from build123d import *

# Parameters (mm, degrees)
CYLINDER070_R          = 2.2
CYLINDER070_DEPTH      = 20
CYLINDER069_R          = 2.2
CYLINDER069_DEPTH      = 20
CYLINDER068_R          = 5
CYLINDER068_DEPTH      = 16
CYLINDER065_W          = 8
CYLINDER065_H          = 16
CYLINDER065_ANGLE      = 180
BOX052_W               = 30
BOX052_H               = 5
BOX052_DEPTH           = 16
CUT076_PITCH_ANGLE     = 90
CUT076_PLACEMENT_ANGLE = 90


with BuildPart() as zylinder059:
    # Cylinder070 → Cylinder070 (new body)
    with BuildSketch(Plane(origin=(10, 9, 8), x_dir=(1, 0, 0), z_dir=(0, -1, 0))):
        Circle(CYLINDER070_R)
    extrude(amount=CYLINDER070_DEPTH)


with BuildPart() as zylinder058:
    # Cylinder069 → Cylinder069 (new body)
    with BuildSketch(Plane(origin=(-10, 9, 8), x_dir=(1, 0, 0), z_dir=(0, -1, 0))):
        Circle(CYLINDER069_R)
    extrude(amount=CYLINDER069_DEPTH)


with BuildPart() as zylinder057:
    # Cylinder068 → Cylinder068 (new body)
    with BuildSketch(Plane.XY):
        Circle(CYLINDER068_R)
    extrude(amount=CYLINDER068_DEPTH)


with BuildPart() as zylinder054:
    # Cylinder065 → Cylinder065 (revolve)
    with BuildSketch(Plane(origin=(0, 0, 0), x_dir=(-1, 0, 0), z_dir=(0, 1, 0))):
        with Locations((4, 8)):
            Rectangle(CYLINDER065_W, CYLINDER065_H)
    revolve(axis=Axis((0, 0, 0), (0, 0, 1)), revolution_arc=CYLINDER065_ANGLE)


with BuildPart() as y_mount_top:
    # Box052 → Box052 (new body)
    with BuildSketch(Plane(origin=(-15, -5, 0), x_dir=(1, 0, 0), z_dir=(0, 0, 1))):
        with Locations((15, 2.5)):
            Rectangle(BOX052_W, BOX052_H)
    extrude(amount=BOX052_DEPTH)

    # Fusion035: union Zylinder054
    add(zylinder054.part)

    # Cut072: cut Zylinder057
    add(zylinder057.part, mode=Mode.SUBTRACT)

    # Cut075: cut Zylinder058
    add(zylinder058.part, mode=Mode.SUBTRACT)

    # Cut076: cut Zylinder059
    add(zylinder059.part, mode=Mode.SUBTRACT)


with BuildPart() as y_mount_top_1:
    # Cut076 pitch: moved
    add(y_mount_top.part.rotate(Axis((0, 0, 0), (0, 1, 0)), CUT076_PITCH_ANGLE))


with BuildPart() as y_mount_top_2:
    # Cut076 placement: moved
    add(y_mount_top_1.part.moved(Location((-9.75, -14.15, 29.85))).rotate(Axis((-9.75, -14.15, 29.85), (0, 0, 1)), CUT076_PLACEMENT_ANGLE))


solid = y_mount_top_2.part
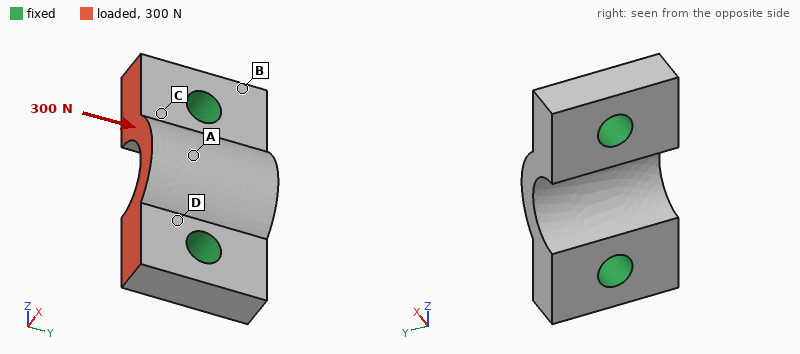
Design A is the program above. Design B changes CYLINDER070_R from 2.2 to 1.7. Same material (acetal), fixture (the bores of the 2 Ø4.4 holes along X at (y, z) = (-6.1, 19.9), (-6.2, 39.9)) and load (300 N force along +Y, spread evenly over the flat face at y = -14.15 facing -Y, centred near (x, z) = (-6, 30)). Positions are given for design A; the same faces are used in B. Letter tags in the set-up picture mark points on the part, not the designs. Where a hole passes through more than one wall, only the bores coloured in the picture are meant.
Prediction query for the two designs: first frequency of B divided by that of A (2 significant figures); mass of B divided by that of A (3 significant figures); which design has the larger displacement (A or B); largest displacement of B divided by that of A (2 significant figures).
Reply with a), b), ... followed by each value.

a) 0.93
b) 1.02
c) B
d) 1.1
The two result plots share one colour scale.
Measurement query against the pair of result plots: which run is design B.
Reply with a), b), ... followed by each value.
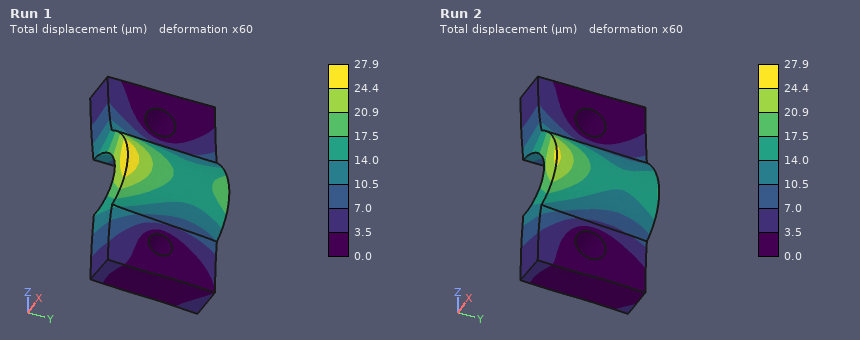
a) Run 1
